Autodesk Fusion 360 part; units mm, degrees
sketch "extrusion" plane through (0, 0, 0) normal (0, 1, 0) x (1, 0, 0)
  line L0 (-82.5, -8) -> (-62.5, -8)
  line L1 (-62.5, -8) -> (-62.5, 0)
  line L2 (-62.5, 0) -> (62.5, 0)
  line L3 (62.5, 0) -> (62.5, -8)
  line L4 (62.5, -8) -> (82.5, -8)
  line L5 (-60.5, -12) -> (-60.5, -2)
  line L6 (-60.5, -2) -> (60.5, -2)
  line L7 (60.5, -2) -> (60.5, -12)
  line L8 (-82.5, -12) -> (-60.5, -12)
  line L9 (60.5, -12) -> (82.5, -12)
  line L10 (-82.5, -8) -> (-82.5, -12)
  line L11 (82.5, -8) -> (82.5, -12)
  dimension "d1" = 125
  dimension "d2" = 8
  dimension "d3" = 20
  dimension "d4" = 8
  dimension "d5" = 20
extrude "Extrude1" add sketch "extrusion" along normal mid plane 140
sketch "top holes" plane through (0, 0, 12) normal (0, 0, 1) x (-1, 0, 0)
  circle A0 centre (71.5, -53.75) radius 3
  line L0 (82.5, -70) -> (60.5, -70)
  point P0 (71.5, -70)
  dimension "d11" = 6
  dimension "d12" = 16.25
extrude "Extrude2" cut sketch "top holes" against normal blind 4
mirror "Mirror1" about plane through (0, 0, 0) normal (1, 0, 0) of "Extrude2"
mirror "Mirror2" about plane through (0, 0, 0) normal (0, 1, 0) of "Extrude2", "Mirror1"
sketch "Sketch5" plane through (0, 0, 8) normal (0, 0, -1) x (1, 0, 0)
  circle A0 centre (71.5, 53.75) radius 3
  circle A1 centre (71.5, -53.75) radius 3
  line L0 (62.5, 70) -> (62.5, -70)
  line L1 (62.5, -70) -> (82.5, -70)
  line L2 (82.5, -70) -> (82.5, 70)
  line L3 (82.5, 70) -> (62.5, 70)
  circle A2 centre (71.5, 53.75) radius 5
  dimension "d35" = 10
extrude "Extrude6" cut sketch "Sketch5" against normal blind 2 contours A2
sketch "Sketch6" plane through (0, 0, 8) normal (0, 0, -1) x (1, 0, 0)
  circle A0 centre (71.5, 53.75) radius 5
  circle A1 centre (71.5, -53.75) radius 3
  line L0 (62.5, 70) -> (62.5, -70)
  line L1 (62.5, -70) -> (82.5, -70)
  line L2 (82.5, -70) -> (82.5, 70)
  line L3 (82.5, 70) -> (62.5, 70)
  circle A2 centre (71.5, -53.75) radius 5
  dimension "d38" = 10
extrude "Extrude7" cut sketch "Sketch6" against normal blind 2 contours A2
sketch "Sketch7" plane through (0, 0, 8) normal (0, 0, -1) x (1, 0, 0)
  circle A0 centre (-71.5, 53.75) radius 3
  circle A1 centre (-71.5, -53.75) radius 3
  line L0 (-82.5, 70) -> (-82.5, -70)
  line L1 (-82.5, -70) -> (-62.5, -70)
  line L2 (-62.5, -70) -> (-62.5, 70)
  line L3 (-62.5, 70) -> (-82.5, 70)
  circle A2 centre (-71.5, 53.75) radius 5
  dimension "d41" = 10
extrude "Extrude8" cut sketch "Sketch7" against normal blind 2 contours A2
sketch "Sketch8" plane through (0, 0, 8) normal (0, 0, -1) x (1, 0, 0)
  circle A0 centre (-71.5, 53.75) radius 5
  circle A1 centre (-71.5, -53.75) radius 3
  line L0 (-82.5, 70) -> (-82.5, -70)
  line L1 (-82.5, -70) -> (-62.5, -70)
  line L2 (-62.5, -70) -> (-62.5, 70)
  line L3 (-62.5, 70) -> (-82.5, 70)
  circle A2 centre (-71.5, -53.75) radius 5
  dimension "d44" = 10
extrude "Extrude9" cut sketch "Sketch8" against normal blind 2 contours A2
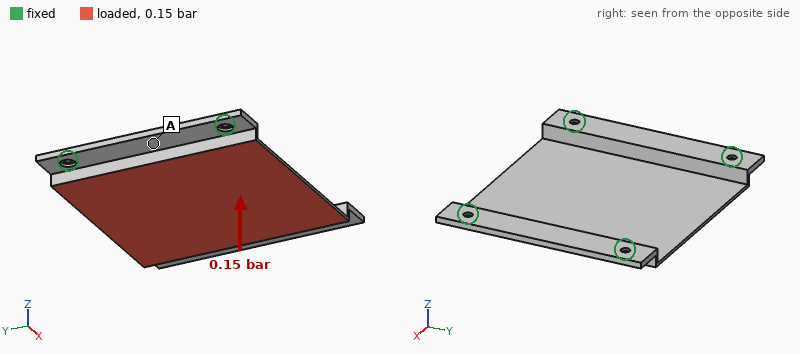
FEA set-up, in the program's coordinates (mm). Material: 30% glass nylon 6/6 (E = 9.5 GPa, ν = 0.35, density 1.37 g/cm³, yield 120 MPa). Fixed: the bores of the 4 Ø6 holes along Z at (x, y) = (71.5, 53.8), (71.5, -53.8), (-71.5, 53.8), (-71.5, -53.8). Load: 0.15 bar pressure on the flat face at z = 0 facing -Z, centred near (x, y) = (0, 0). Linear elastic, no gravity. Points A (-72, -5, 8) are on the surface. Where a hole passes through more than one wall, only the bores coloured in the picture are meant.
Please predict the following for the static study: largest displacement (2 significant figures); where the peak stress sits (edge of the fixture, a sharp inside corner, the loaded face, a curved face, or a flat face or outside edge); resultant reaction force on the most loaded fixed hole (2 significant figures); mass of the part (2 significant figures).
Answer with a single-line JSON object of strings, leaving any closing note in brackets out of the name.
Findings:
{"largest displacement": "1.6 mm", "where the peak stress sits": "the loaded face", "resultant reaction force on the most loaded fixed hole": "210 N", "mass of the part": "85 g"}
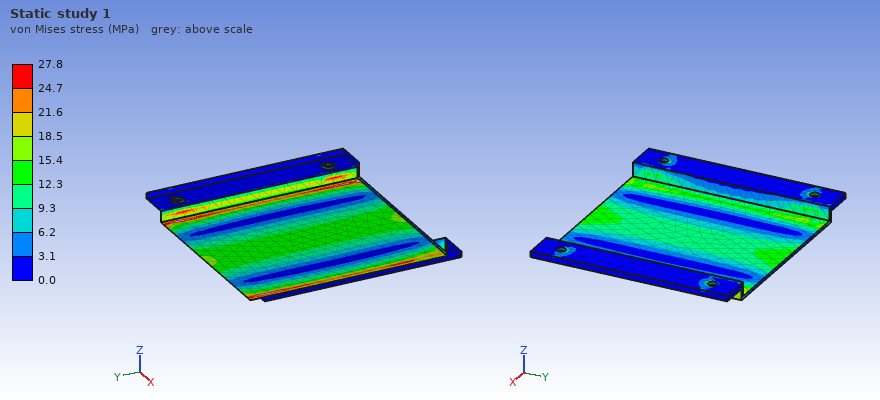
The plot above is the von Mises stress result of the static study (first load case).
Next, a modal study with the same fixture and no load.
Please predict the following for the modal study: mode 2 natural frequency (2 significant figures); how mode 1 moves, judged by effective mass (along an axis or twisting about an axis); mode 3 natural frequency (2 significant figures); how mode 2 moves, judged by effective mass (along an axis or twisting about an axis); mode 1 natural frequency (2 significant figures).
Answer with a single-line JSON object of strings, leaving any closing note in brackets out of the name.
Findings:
{"mode 2 natural frequency": "410 Hz", "how mode 1 moves, judged by effective mass": "along Z", "mode 3 natural frequency": "620 Hz", "how mode 2 moves, judged by effective mass": "twisting about X", "mode 1 natural frequency": "350 Hz"}
